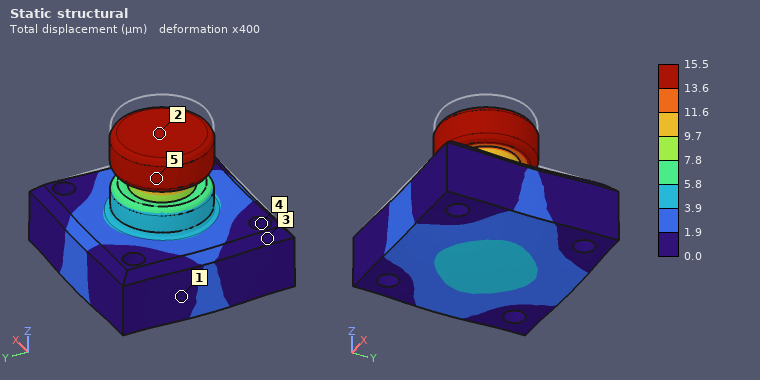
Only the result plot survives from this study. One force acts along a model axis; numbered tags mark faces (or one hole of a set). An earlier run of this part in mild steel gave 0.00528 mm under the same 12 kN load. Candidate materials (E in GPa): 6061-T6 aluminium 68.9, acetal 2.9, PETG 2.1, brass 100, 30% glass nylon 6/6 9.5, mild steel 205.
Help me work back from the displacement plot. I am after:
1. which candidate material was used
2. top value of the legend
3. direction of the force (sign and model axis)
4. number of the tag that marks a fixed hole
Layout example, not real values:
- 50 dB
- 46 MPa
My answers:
- 6061-T6 aluminium
- 15.5 µm
- -Z
- 4
